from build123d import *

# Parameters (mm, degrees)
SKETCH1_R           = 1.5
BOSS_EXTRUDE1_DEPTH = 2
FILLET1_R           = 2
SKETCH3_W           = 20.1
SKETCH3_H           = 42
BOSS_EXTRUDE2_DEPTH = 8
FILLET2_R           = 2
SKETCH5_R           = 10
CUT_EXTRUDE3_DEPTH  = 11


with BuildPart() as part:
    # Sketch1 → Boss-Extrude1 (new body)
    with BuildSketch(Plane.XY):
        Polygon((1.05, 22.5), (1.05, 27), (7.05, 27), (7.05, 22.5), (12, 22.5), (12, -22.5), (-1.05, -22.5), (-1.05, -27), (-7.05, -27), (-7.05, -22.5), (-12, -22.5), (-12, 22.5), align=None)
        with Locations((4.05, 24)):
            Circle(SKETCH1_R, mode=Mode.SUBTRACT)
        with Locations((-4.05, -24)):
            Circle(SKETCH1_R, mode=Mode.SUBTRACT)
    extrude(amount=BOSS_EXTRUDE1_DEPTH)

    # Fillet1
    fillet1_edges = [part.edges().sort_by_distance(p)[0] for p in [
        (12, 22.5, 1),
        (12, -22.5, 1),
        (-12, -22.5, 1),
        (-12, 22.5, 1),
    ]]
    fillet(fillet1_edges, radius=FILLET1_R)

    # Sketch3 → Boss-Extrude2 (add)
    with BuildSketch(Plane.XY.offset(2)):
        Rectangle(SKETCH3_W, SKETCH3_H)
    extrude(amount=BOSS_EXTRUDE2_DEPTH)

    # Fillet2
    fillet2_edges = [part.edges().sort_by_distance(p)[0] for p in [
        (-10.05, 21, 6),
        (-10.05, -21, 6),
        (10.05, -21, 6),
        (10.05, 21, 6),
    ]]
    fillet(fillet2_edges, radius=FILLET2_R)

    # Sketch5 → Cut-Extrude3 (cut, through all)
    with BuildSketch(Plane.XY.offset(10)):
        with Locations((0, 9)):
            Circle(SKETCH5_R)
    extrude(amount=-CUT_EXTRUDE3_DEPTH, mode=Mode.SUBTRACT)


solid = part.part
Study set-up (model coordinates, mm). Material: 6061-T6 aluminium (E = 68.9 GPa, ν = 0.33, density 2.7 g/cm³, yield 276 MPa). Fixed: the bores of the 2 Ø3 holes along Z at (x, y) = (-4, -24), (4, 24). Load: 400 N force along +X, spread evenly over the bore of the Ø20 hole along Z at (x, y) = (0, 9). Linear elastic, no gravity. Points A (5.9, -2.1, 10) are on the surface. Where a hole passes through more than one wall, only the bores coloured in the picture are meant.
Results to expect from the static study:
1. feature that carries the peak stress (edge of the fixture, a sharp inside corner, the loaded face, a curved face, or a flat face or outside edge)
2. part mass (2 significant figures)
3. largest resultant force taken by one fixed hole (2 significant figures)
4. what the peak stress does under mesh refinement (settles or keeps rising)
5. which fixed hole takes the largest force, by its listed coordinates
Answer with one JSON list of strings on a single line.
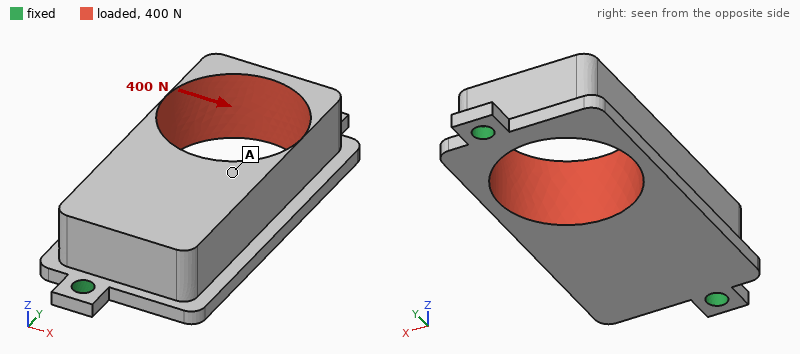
["edge of the fixture", "16 g", "270 N", "keeps rising", "(4, 24)"]
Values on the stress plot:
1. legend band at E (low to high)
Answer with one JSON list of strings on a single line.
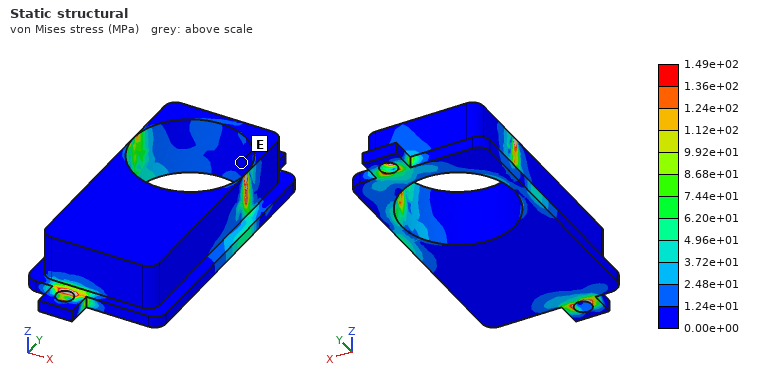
["0.00e+00 to 1.24e+01 MPa"]
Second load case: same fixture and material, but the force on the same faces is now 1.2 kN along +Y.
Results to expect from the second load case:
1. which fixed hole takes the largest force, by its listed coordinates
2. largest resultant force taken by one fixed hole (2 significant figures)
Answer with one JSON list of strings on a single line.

["(-4, -24)", "750 N"]
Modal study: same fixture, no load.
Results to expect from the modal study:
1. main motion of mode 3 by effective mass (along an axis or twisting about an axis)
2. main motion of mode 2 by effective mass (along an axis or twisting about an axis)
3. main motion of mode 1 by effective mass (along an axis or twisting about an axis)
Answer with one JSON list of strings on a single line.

["along X", "along Z", "along X"]
